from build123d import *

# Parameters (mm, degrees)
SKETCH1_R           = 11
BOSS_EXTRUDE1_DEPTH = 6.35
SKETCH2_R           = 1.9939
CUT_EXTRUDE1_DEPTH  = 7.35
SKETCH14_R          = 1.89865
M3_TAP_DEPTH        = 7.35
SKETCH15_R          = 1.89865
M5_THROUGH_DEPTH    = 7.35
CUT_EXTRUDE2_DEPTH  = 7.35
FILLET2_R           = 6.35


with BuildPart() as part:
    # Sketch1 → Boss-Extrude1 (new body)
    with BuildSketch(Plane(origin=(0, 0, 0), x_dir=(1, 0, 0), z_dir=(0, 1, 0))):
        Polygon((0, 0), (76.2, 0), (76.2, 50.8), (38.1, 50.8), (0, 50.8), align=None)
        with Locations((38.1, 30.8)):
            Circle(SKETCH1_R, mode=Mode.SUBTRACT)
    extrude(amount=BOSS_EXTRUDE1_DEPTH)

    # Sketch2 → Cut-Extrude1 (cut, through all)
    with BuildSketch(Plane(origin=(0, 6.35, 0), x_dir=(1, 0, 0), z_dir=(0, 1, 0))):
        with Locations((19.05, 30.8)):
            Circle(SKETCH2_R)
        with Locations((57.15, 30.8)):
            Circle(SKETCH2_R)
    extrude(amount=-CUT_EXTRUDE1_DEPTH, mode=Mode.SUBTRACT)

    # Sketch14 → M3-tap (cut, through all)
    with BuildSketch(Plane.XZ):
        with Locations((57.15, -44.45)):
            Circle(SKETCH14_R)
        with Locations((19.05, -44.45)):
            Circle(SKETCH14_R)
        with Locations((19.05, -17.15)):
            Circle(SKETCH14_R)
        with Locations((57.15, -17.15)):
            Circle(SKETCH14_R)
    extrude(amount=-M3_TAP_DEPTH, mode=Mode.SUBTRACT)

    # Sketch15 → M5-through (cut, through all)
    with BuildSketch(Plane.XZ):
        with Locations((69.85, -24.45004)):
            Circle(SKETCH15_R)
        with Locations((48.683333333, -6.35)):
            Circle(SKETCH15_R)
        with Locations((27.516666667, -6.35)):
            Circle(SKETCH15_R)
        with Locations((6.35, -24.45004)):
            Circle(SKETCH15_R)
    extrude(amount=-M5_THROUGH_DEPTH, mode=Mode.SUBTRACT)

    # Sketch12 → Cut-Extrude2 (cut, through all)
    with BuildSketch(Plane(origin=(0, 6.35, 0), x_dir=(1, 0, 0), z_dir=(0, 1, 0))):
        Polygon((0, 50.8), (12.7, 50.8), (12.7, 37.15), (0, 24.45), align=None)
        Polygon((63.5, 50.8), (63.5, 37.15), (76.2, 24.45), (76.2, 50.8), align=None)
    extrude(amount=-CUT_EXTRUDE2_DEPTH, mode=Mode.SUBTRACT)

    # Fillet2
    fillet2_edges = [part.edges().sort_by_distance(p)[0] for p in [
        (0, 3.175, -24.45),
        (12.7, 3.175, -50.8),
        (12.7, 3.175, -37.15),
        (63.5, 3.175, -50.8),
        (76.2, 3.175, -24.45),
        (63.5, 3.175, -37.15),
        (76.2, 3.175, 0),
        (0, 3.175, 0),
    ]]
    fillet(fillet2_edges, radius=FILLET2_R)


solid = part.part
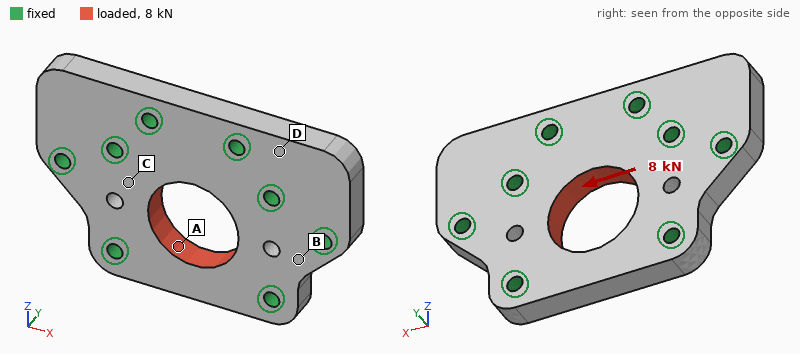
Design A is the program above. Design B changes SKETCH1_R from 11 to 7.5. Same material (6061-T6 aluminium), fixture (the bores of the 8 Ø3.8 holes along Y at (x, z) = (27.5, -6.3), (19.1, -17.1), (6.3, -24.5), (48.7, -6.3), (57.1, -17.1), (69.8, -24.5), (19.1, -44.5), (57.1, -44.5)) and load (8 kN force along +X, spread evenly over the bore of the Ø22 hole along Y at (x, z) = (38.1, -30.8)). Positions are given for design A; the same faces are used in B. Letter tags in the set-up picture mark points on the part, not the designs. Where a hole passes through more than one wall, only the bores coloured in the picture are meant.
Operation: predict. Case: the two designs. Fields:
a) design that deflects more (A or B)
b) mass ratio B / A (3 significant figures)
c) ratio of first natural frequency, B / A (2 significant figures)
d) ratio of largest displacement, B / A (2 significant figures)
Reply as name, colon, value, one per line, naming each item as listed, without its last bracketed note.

design that deflects more: B
mass ratio B / A: 1.07
ratio of first natural frequency, B / A: 1.00
ratio of largest displacement, B / A: 1.3
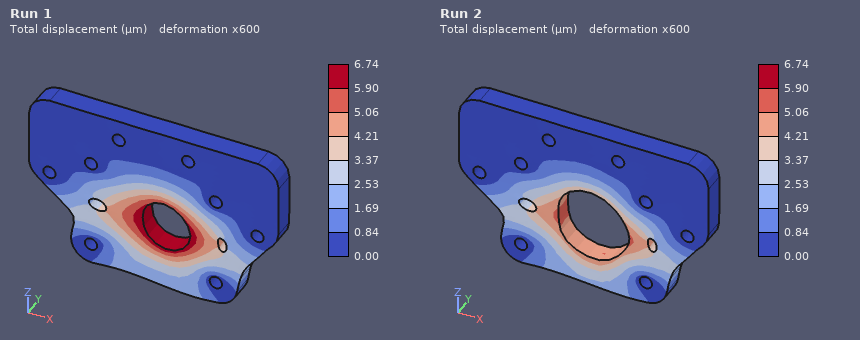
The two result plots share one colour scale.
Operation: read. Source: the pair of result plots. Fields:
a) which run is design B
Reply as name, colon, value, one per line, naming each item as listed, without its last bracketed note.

which run is design B: Run 1
